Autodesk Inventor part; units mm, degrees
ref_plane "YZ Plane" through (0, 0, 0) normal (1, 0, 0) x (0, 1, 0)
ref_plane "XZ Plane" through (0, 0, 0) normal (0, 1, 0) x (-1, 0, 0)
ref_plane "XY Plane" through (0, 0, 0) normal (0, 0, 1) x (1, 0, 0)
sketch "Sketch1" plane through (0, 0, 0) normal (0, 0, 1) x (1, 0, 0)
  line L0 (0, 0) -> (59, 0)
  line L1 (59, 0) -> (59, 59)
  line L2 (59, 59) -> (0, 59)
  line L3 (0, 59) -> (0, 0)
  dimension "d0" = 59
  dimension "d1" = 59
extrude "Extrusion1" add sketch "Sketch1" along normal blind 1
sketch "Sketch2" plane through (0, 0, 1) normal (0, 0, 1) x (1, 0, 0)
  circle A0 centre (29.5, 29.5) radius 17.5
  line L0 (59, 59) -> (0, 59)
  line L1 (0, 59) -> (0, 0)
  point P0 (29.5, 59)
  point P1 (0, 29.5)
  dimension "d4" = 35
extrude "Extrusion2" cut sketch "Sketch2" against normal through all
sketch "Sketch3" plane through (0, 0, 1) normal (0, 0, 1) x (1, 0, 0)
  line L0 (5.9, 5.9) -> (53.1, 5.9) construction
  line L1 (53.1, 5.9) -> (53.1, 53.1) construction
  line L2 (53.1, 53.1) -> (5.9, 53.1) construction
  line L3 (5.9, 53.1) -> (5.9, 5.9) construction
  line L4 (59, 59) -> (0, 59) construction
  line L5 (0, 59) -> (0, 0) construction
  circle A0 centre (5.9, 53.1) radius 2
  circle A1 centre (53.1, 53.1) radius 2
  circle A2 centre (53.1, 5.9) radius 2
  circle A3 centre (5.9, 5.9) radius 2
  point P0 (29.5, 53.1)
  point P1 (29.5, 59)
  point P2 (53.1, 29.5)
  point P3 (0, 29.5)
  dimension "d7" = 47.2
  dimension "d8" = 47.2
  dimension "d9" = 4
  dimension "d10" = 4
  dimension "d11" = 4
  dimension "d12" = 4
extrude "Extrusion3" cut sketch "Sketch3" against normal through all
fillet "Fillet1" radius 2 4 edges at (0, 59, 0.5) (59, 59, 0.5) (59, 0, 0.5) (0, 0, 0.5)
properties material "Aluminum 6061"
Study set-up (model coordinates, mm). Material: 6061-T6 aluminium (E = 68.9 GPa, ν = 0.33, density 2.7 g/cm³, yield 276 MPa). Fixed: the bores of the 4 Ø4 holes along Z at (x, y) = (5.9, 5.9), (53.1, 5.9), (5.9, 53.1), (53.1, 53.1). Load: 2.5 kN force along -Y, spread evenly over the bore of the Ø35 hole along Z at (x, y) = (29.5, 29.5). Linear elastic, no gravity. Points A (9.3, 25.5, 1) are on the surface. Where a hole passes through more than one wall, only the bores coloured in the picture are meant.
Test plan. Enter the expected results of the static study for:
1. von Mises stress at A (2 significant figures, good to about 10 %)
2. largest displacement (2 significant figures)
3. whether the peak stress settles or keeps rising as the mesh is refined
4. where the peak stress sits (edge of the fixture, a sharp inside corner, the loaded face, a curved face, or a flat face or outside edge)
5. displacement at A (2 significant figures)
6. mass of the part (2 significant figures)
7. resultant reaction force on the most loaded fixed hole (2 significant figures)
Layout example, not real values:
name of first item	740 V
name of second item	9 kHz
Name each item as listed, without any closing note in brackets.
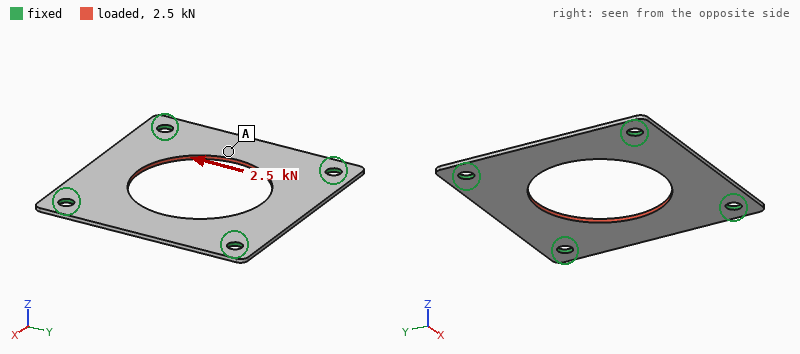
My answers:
von Mises stress at A	46 MPa
largest displacement	31 µm
whether the peak stress settles or keeps rising as the mesh is refined	keeps rising
where the peak stress sits	edge of the fixture
displacement at A	10 µm
mass of the part	6.7 g
resultant reaction force on the most loaded fixed hole	650 N
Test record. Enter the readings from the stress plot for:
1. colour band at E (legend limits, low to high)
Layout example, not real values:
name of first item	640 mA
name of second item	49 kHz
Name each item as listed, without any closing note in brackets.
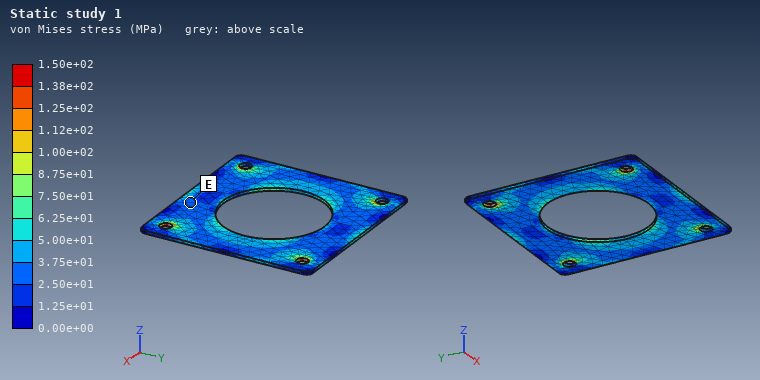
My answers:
colour band at E	2.50e+01 to 3.75e+01 MPa
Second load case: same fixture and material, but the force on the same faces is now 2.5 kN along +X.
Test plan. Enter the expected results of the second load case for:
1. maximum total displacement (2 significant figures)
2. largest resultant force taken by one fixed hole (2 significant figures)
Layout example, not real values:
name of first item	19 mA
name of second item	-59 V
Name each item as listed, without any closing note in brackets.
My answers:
maximum total displacement	31 µm
largest resultant force taken by one fixed hole	650 N
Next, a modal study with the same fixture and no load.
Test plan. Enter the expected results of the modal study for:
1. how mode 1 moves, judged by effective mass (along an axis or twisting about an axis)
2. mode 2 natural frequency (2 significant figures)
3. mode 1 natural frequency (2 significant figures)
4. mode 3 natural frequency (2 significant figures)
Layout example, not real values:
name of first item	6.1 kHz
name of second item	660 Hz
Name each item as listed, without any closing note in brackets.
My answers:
how mode 1 moves, judged by effective mass	along Z
mode 2 natural frequency	2800 Hz
mode 1 natural frequency	2600 Hz
mode 3 natural frequency	2800 Hz
